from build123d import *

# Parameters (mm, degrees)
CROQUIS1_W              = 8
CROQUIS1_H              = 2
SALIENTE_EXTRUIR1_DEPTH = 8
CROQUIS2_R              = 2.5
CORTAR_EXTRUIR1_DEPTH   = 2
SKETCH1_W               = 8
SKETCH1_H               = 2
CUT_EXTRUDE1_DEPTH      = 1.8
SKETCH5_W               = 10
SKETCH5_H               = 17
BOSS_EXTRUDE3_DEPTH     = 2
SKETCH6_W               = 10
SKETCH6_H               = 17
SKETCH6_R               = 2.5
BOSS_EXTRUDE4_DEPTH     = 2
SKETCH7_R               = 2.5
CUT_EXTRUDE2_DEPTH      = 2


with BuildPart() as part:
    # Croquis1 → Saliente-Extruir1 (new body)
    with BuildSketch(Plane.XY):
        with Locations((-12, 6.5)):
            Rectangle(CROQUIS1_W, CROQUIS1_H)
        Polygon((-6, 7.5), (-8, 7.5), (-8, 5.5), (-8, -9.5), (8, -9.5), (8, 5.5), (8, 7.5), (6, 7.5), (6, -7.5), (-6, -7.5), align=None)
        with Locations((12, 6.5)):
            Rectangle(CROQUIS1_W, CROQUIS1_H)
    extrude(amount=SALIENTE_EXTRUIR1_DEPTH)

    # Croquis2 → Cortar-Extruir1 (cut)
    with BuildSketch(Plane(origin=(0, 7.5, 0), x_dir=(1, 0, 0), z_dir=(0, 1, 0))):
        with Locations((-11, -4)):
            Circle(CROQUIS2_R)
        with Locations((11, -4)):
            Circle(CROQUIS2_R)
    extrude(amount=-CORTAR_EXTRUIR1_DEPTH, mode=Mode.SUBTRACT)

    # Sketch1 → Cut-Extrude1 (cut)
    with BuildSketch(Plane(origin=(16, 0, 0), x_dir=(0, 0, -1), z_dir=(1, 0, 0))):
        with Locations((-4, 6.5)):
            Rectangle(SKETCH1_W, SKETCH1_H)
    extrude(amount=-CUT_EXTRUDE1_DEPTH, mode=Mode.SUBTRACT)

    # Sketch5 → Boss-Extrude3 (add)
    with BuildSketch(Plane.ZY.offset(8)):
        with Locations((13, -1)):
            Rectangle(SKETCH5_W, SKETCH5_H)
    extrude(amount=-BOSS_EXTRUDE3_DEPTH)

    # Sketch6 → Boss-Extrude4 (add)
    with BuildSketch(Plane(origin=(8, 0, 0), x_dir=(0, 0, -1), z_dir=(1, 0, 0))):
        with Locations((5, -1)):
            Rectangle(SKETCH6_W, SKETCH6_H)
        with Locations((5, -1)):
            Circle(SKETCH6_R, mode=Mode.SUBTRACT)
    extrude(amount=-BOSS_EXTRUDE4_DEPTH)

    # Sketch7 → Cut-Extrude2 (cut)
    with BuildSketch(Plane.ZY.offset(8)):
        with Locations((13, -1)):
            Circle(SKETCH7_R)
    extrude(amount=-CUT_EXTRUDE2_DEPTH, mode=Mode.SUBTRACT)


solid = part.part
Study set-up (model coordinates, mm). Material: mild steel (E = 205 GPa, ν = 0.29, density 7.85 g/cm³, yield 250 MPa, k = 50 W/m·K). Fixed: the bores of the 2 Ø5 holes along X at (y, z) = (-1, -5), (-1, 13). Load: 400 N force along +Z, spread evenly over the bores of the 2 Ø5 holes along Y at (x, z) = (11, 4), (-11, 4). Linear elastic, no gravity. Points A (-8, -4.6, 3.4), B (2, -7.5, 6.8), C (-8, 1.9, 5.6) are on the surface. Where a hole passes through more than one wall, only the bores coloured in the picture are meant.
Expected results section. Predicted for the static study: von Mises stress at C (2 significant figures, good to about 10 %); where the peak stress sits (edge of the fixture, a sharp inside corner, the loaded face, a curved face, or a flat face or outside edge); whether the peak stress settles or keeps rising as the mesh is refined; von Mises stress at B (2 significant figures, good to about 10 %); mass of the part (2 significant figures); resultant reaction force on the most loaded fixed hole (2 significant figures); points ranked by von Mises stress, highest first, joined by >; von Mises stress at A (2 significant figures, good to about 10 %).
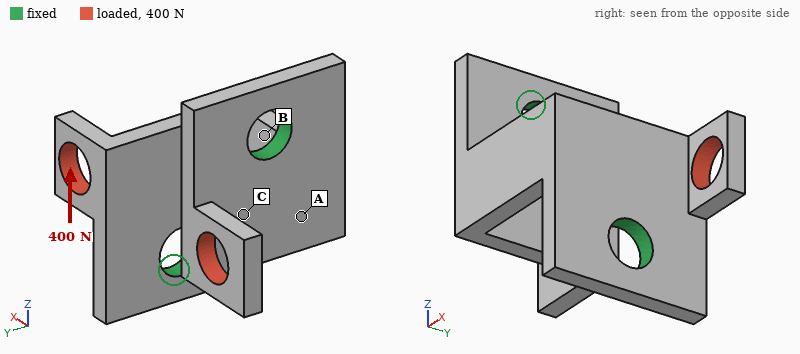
69 MPa
a sharp inside corner
keeps rising
19 MPa
12 g
200 N
C > A > B
45 MPa
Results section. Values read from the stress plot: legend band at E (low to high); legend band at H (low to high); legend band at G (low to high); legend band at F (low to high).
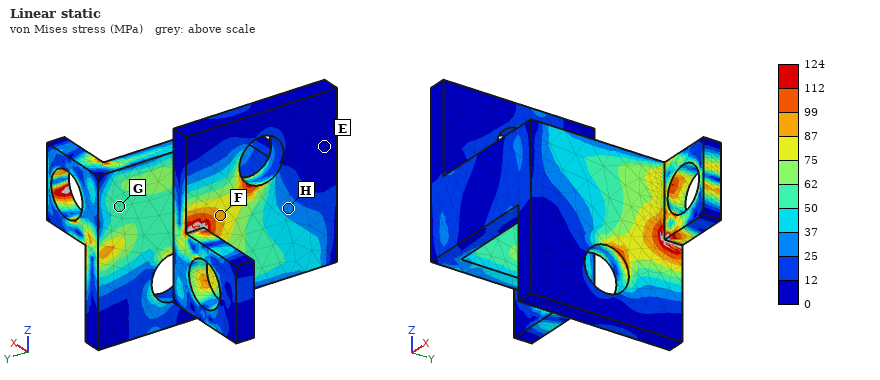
0 to 12 MPa
25 to 37 MPa
50 to 62 MPa
87 to 99 MPa
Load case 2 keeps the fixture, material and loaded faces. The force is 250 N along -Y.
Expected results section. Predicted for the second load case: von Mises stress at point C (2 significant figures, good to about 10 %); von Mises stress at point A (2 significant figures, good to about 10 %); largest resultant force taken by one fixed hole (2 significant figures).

52 MPa
13 MPa
130 N
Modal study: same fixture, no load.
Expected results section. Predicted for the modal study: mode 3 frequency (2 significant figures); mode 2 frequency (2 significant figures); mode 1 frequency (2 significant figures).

12 kHz
10 kHz
8300 Hz
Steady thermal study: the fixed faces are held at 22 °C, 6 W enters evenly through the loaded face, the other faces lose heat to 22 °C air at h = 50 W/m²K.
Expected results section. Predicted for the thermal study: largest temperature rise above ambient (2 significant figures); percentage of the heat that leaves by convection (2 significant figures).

50 K
16 %
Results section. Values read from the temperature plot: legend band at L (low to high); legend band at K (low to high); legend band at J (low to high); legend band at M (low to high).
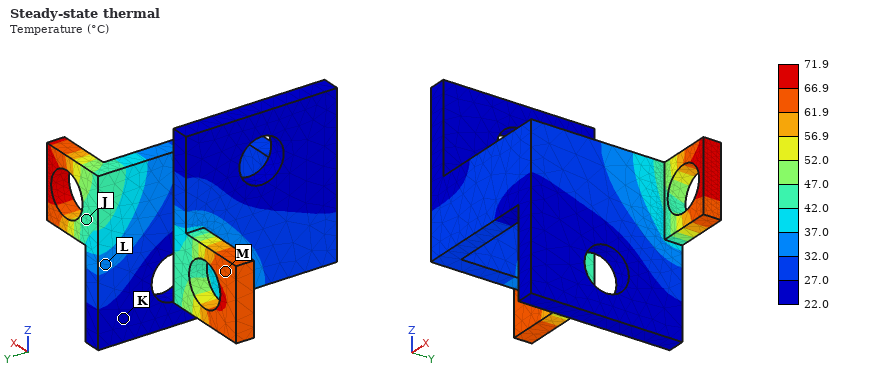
32.0 to 37.0 °C
22.0 to 27.0 °C
42.0 to 47.0 °C
61.9 to 66.9 °C
